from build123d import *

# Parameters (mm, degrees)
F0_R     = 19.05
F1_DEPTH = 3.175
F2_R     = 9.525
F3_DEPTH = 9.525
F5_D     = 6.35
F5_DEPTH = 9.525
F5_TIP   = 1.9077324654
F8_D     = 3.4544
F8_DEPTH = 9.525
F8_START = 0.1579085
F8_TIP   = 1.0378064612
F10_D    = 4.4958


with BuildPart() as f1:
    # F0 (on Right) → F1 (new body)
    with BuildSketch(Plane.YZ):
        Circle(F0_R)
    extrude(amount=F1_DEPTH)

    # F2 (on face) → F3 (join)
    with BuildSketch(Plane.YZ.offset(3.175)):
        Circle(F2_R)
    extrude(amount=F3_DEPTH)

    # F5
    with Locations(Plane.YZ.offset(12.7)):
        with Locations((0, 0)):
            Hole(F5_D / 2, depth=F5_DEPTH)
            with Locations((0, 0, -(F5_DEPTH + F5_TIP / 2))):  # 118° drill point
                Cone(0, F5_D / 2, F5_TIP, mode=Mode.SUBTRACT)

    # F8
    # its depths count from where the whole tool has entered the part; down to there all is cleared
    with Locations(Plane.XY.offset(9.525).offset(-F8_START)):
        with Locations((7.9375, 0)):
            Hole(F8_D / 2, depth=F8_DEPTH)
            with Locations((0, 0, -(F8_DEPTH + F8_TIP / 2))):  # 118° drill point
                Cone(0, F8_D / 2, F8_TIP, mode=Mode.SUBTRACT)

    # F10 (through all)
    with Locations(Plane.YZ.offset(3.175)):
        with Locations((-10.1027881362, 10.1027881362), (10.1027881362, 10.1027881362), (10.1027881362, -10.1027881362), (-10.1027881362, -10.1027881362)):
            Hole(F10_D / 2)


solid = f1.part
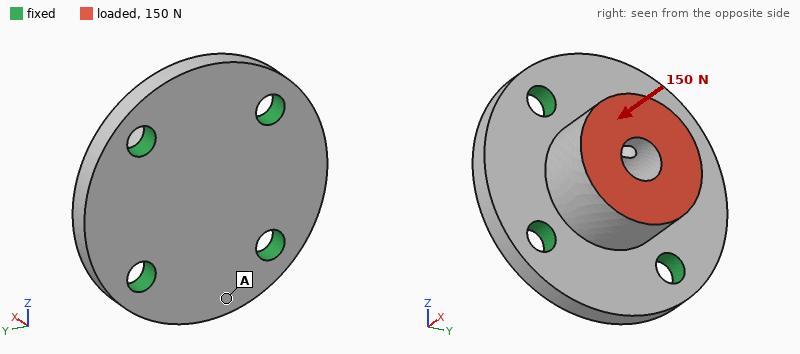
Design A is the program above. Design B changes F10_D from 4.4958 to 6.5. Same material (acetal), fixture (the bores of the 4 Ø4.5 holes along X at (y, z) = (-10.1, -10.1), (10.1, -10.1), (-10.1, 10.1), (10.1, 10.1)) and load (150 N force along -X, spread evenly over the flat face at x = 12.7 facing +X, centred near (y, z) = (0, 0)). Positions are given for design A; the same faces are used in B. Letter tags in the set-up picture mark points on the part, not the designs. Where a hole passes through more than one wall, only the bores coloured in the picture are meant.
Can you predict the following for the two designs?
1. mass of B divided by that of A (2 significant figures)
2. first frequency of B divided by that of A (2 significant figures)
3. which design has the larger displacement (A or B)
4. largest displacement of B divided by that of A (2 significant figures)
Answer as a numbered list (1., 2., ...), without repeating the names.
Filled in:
1. 0.96
2. 1.2
3. A
4. 0.71
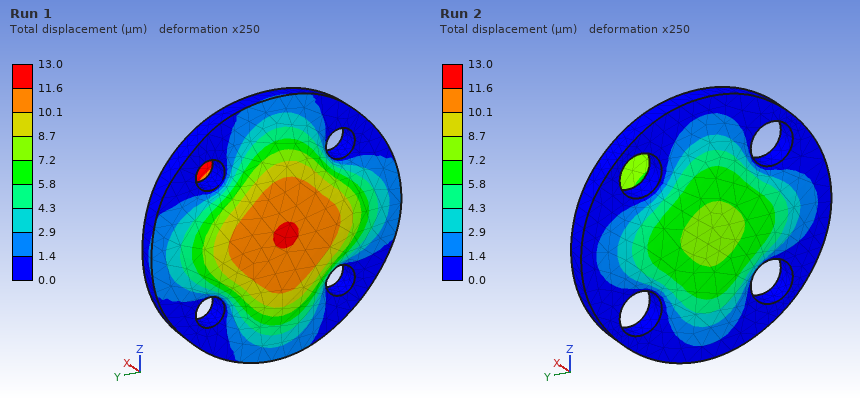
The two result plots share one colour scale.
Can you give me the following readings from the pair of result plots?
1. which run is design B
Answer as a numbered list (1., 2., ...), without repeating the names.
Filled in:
1. Run 2
